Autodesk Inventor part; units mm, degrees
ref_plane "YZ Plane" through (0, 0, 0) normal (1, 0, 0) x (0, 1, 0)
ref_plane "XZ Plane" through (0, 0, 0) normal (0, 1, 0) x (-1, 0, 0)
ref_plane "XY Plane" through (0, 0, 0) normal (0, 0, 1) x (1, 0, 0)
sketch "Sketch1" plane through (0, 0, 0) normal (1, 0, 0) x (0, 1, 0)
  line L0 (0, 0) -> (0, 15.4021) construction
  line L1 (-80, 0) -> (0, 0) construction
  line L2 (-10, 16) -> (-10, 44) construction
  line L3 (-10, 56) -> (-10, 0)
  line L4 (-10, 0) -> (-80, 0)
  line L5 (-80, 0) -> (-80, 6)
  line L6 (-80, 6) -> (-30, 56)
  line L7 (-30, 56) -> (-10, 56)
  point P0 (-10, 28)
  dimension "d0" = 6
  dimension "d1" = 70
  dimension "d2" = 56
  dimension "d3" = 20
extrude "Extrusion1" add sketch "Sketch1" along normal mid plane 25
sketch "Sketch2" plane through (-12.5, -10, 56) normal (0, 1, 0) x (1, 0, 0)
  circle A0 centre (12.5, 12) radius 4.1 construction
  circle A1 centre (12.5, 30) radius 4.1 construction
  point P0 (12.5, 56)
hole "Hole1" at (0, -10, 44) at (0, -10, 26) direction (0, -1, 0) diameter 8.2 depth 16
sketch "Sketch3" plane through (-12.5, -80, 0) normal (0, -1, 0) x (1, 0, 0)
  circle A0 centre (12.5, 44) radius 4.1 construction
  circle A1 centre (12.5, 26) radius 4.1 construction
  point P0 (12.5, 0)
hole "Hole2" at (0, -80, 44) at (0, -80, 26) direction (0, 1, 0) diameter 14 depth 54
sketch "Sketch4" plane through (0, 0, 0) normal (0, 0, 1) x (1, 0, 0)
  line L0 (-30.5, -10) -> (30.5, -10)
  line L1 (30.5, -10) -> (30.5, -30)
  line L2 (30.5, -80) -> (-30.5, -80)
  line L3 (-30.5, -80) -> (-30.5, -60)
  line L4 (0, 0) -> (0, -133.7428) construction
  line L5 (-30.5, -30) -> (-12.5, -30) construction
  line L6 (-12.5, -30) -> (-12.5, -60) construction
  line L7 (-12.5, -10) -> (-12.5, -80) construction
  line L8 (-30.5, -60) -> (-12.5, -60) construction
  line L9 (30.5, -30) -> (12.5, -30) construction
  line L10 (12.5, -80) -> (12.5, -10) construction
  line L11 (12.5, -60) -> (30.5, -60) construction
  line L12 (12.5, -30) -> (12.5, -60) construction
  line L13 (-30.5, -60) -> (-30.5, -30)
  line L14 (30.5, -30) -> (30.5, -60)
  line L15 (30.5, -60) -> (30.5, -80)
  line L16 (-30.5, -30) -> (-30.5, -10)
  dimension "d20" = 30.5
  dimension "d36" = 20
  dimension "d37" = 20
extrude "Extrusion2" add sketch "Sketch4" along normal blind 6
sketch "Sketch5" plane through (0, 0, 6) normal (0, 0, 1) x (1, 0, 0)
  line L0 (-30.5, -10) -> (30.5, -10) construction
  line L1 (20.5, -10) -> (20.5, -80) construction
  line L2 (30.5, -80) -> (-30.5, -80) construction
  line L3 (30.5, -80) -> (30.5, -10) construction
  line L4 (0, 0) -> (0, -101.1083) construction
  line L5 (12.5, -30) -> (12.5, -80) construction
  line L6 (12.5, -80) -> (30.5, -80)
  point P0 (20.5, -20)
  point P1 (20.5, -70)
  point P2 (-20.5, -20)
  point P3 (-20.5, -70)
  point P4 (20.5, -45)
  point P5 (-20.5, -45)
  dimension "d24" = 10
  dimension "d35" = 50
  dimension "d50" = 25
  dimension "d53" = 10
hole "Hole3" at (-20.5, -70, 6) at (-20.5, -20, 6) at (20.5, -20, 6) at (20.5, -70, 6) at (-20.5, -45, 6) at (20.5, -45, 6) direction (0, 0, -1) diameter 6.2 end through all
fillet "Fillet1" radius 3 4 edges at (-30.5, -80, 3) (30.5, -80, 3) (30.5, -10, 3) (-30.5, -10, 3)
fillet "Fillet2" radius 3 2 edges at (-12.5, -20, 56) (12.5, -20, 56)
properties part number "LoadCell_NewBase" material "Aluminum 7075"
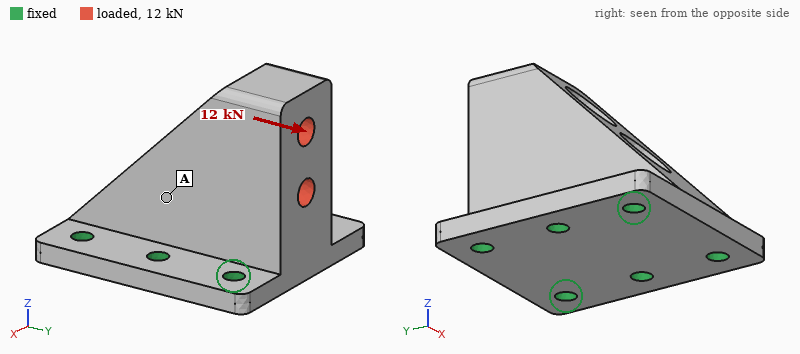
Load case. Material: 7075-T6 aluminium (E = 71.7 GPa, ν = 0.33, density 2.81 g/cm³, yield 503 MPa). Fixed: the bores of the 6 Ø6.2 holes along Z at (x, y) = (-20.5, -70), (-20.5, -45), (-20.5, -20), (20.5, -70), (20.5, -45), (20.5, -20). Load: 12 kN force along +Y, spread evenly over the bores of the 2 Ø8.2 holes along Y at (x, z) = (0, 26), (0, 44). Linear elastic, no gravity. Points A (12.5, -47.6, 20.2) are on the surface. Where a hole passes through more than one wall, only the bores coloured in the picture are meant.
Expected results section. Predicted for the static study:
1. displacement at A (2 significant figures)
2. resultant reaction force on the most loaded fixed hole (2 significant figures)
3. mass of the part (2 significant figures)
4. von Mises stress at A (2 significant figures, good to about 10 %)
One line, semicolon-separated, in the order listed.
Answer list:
0.029 mm; 4.7 kN; 200 g; 25 MPa
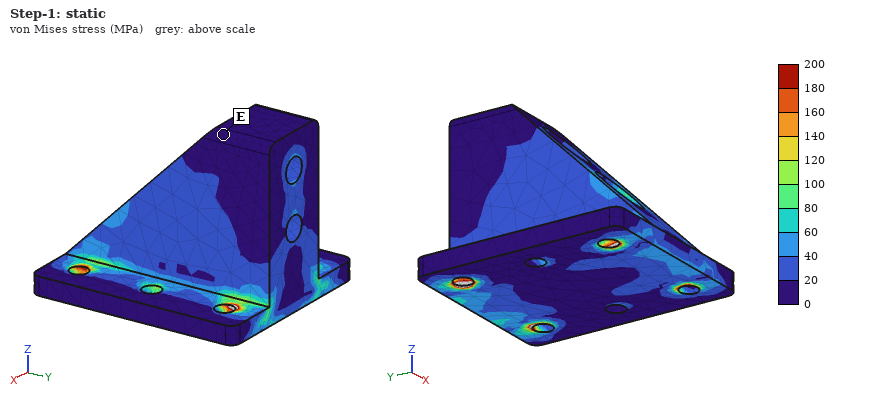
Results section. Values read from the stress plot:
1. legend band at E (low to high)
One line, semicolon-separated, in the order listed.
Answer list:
0 to 20 MPa
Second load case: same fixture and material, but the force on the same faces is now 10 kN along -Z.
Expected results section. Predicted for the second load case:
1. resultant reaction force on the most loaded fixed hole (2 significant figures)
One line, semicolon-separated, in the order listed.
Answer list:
4.6 kN
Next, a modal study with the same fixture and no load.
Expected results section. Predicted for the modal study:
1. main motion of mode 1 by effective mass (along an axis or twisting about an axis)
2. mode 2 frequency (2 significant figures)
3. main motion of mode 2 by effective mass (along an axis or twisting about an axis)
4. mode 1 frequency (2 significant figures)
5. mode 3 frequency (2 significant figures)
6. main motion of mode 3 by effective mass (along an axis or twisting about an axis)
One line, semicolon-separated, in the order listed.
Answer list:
along X; 6600 Hz; along Y; 5500 Hz; 12 kHz; along Z
